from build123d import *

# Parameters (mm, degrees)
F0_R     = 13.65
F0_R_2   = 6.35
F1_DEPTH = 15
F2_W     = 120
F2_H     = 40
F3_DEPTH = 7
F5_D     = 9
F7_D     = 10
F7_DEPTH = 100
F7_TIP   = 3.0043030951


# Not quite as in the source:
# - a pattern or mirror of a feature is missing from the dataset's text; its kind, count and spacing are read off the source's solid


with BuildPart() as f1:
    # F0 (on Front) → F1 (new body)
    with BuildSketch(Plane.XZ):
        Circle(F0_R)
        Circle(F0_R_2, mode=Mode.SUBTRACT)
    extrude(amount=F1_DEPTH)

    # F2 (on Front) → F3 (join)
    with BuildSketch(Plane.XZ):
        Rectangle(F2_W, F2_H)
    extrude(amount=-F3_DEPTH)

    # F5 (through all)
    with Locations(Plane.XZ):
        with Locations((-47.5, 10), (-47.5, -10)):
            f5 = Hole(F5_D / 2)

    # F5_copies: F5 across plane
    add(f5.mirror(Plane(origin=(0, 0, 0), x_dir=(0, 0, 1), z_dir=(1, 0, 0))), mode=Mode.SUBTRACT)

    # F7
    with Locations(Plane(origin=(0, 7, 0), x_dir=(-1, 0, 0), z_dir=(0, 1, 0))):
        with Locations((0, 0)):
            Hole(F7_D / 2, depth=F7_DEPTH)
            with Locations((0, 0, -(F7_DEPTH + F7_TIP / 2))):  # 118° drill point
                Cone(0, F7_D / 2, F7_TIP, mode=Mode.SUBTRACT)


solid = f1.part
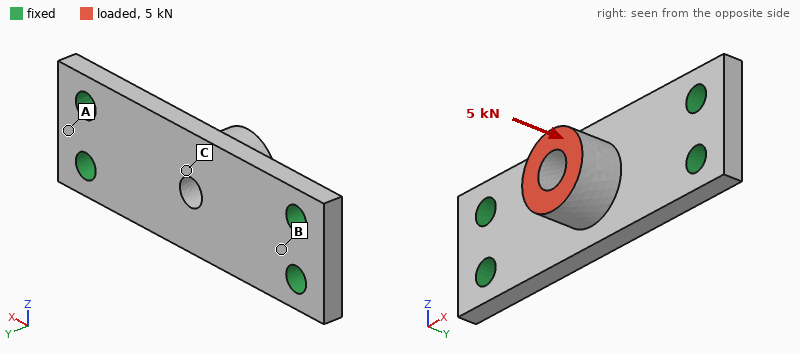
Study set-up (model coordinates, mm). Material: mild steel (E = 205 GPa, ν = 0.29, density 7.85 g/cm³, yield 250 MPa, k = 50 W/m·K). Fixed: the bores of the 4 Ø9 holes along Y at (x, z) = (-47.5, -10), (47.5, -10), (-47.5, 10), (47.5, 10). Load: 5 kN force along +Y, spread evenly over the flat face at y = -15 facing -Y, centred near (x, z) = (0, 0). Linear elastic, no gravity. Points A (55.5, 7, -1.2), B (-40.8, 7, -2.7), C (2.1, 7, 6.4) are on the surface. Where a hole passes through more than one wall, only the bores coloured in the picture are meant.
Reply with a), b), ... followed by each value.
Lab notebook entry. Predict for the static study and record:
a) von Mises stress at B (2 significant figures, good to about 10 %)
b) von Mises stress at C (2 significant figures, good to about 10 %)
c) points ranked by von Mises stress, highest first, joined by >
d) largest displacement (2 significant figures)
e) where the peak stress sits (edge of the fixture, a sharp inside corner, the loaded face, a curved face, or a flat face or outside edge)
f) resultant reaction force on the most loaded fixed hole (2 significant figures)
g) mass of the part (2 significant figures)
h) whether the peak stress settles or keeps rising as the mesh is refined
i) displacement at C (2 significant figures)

a) 88 MPa
b) 58 MPa
c) B > C > A
d) 54 µm
e) edge of the fixture
f) 1.4 kN
g) 300 g
h) keeps rising
i) 53 µm
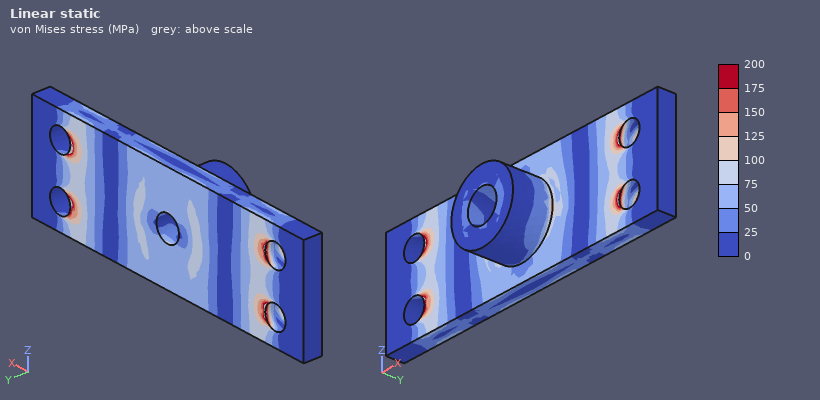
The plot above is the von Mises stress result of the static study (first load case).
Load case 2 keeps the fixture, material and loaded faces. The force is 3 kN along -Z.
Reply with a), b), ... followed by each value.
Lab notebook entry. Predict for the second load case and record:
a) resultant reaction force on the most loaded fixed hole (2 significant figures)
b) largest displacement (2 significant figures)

a) 1.7 kN
b) 54 µm
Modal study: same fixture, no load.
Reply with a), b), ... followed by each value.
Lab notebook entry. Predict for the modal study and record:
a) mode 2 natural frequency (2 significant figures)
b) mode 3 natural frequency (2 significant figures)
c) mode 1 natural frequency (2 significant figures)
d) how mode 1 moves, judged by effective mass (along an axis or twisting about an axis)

a) 5400 Hz
b) 9400 Hz
c) 4100 Hz
d) along Y
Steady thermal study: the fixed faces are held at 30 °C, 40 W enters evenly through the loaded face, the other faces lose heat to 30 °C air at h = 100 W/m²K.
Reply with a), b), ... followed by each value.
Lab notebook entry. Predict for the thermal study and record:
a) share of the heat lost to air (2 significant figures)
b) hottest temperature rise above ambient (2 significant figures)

a) 52 %
b) 55 K
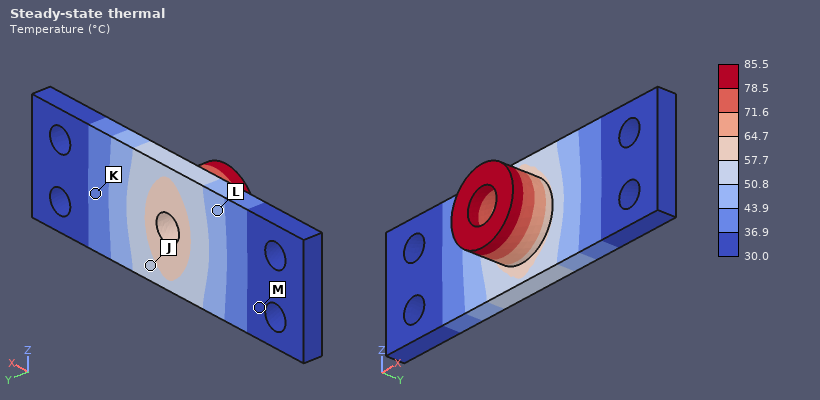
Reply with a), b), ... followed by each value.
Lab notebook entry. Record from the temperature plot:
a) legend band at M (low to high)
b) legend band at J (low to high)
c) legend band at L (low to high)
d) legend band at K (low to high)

a) 30.0 to 36.9 °C
b) 50.8 to 57.7 °C
c) 43.9 to 50.8 °C
d) 36.9 to 43.9 °C
